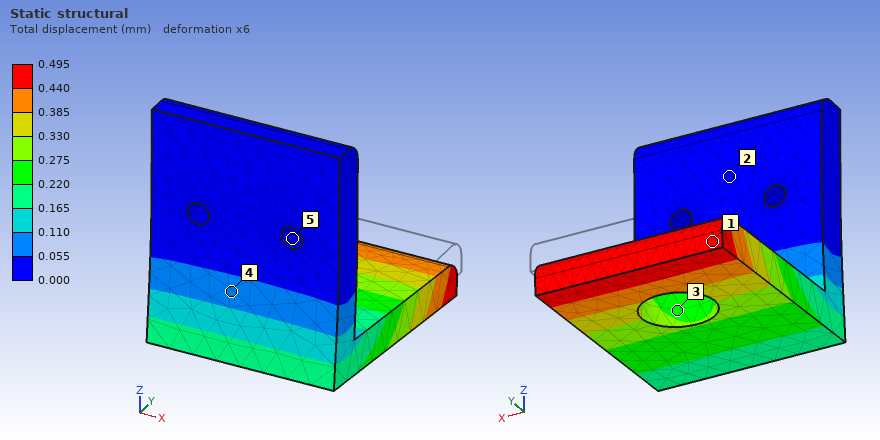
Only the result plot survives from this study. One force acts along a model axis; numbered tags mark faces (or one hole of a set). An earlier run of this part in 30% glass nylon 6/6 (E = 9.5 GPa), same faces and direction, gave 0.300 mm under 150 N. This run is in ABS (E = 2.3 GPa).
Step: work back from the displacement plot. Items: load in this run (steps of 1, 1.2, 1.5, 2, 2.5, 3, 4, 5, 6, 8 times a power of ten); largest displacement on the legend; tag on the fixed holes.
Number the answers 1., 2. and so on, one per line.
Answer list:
1. 60 N
2. 0.495 mm
3. 5
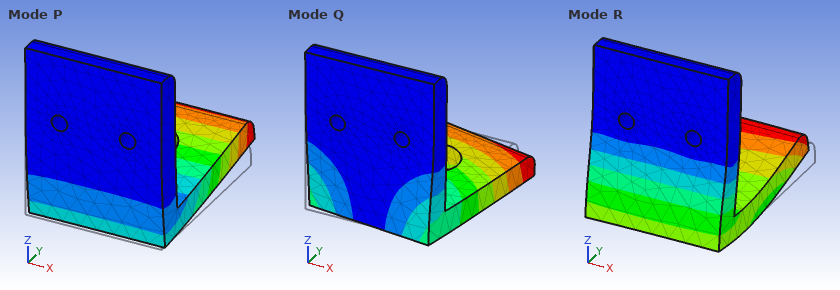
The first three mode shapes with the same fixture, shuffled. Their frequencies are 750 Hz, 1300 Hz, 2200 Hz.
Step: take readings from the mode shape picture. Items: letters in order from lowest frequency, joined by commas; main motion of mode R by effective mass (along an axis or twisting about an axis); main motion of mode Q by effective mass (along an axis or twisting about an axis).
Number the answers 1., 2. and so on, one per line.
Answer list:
1. P, Q, R
2. along Y
3. along X
